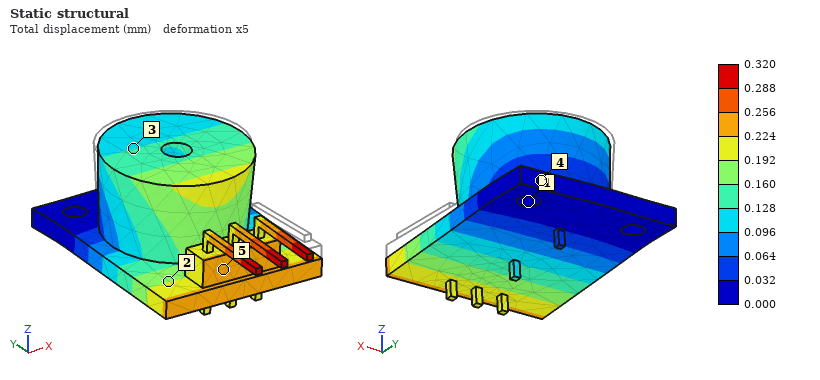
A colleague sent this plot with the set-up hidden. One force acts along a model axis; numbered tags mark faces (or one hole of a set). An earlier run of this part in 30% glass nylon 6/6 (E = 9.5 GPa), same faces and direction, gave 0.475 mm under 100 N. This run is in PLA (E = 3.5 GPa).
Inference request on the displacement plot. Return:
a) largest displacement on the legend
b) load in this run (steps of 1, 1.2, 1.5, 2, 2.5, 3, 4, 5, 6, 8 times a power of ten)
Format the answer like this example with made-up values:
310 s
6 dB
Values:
0.320 mm
25 N
